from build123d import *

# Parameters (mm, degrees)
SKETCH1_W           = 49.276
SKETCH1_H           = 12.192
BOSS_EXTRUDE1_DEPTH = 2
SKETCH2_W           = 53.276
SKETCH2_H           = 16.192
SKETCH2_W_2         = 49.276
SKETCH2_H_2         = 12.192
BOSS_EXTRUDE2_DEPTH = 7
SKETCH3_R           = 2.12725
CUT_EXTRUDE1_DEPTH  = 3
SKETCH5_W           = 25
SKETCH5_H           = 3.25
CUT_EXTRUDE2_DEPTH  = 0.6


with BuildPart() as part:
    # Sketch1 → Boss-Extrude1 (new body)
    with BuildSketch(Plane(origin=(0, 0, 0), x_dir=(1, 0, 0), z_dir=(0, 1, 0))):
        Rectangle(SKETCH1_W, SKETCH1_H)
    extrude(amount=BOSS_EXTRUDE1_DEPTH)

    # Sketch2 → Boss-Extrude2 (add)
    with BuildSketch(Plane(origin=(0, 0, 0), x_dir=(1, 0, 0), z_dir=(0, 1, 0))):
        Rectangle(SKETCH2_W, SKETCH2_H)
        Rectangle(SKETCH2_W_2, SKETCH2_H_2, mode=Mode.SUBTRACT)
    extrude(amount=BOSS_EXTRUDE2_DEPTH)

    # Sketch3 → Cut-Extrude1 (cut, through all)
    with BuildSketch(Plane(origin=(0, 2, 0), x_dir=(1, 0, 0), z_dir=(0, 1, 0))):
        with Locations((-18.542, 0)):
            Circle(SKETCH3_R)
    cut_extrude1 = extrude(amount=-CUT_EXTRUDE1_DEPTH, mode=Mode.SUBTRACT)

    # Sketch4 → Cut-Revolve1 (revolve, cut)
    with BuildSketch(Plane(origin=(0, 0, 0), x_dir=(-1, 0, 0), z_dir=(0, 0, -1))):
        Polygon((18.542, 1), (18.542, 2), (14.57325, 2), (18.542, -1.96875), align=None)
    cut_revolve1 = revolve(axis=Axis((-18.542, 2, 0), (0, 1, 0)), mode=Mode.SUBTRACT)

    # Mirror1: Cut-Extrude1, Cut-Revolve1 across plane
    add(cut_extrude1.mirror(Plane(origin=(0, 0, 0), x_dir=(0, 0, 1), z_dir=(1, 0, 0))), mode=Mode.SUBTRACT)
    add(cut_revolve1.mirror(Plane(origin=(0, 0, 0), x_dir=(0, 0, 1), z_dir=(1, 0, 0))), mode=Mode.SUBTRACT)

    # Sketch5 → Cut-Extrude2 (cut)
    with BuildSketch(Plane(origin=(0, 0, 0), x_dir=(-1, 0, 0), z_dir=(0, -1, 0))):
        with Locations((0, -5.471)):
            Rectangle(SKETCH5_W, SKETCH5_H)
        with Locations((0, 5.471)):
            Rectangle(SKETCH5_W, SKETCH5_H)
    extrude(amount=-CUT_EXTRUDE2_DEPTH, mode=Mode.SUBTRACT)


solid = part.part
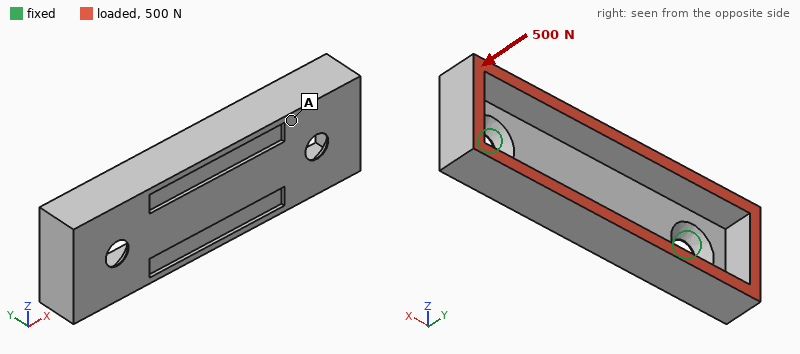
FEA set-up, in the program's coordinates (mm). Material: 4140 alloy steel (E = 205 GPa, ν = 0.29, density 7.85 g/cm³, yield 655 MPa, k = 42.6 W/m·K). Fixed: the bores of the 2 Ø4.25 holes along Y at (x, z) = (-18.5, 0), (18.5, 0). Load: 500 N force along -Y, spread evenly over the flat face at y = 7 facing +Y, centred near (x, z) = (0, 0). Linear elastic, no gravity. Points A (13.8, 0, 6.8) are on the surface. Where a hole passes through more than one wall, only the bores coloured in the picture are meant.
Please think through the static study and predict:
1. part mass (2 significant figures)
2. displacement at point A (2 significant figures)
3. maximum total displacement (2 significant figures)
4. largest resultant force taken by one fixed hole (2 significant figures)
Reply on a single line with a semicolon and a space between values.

22 g; 4.4 µm; 6.9 µm; 260 N
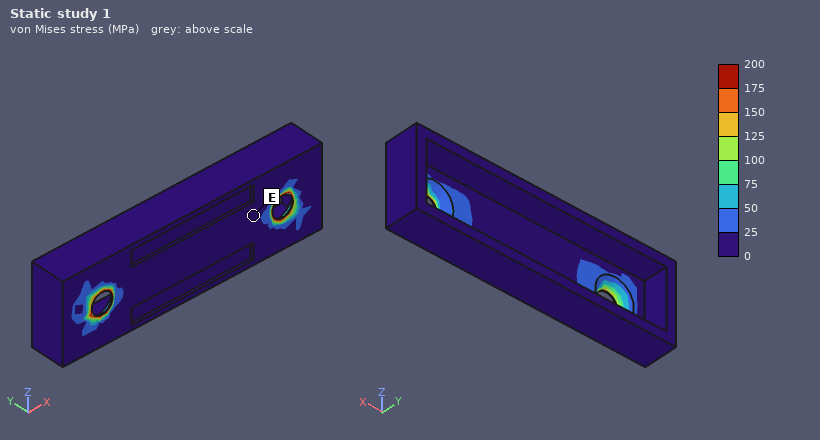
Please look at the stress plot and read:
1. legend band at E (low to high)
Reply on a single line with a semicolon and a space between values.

0 to 25 MPa
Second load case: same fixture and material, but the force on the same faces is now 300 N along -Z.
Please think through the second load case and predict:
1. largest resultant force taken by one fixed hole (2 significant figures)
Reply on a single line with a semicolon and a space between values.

150 N
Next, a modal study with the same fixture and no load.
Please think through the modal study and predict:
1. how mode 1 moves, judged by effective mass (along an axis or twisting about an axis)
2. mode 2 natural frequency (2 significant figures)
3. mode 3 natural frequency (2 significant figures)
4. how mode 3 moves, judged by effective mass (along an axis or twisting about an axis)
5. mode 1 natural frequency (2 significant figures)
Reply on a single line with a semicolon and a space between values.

along Z; 7000 Hz; 10 kHz; along Y; 4200 Hz
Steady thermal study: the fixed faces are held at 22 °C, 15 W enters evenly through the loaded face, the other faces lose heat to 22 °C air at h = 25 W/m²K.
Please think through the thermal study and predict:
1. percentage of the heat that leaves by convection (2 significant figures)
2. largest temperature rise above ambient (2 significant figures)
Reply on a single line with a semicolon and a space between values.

19 %; 48 K
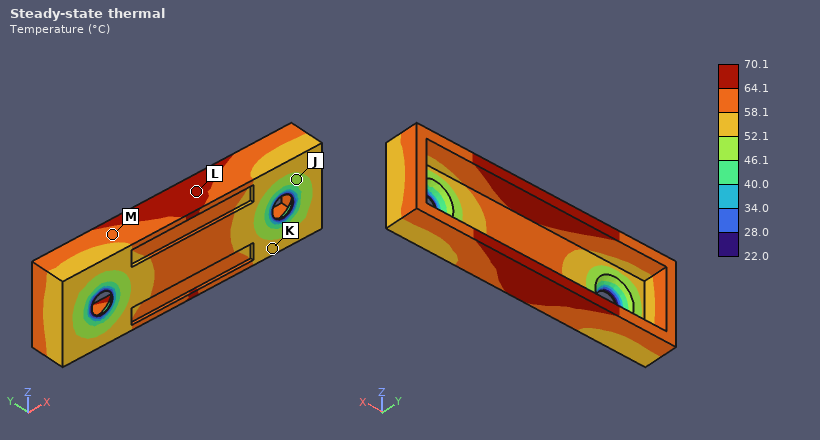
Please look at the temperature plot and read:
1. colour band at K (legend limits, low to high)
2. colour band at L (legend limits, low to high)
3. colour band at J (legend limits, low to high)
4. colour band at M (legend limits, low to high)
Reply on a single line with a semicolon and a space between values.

52.1 to 58.1 °C; 64.1 to 70.1 °C; 46.1 to 52.1 °C; 58.1 to 64.1 °C
